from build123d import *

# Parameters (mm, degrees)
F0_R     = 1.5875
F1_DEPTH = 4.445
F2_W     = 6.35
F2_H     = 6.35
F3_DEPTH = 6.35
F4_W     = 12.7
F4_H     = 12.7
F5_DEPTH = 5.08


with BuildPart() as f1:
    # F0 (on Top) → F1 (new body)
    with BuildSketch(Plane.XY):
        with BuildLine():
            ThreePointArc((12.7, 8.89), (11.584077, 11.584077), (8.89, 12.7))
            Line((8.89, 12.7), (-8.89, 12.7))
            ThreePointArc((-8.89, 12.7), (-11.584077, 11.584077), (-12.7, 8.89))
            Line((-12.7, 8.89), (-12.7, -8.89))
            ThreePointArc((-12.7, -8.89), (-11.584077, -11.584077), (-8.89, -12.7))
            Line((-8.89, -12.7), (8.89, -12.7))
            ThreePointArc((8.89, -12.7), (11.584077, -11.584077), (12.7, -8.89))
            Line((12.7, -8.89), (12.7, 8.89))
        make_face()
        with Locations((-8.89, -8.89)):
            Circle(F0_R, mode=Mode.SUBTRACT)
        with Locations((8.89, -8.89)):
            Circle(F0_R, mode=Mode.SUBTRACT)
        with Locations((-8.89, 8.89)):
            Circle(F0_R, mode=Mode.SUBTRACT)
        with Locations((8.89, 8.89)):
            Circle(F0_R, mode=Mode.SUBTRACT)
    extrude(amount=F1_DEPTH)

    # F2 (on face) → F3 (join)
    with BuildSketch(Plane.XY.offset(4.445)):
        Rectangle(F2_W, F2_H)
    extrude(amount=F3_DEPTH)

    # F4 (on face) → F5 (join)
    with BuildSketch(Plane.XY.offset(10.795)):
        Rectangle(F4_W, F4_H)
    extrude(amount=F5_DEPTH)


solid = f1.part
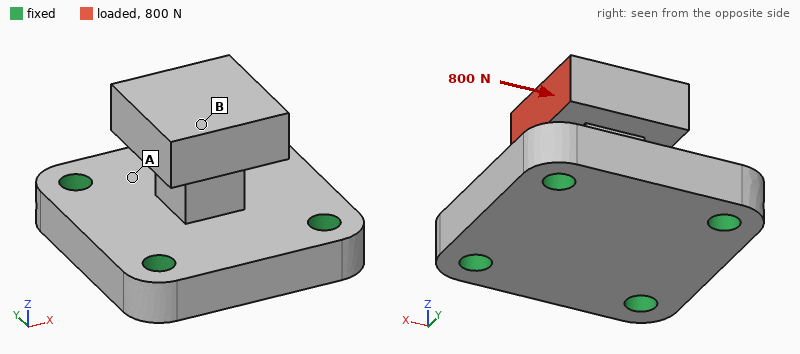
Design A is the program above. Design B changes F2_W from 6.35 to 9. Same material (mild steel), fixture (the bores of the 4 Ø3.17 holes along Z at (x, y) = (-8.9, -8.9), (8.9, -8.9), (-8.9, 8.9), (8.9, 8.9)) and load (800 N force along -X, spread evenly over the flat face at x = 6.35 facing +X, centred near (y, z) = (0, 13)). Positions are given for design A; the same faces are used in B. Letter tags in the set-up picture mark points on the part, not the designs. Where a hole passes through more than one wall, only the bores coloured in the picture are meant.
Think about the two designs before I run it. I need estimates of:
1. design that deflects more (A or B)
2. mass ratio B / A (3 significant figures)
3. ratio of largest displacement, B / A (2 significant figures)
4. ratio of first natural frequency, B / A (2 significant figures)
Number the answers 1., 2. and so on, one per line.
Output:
1. A
2. 1.03
3. 0.50
4. 1.1
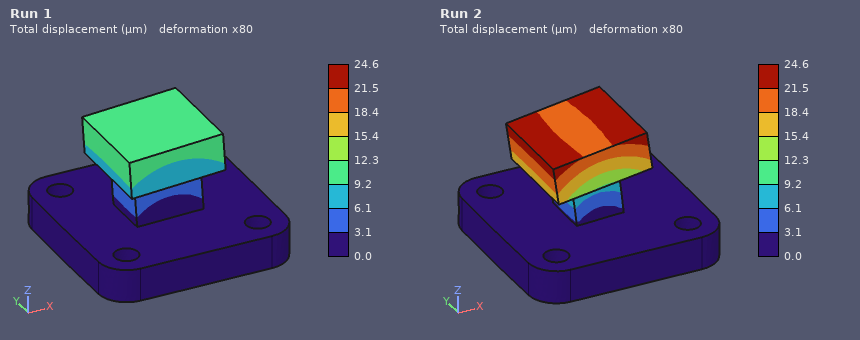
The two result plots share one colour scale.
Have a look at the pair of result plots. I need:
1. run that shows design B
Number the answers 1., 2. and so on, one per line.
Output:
1. Run 1
